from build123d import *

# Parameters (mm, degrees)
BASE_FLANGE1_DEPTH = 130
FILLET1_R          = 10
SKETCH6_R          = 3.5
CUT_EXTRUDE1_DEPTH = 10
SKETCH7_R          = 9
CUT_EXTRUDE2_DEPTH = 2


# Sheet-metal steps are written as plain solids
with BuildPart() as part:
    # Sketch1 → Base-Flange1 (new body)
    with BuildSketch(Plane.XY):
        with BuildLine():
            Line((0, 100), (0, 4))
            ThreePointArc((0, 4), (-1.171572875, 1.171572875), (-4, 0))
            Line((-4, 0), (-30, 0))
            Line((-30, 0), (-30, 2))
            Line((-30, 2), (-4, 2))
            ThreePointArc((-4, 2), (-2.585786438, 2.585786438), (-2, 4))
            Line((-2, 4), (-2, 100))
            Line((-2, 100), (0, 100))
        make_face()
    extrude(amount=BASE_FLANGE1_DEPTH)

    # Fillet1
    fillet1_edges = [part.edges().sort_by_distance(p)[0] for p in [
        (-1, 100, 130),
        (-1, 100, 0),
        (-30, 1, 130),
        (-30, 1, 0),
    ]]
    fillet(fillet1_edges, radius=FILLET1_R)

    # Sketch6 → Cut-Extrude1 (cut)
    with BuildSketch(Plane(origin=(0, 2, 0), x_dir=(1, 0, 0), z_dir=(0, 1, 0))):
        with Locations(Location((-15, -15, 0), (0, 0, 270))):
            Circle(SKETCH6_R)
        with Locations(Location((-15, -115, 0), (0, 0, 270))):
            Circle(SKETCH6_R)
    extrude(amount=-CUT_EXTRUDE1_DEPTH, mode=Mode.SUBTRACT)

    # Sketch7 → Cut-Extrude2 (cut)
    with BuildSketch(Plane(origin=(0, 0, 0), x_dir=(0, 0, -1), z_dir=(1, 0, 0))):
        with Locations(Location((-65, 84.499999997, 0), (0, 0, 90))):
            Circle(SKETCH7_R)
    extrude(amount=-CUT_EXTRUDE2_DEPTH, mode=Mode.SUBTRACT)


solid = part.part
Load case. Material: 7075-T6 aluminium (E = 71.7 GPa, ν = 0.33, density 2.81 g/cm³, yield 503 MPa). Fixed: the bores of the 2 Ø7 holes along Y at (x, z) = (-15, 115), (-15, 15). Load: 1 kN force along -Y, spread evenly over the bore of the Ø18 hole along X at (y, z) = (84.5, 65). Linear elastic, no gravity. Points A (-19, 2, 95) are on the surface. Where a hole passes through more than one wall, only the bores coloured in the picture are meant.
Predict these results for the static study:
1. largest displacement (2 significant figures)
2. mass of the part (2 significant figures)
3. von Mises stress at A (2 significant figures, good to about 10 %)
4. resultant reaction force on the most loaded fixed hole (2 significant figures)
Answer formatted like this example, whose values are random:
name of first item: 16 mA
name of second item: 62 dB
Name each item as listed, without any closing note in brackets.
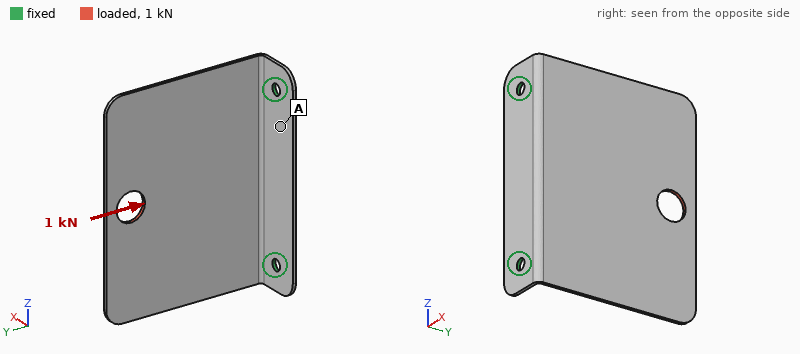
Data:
largest displacement: 1.9 mm
mass of the part: 90 g
von Mises stress at A: 38 MPa
resultant reaction force on the most loaded fixed hole: 510 N
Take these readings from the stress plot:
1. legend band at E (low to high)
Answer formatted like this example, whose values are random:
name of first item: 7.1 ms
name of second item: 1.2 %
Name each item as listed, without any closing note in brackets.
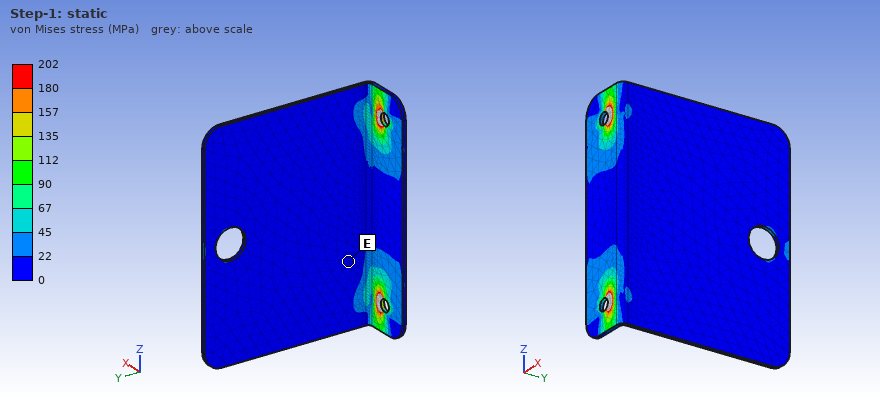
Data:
legend band at E: 0 to 22 MPa
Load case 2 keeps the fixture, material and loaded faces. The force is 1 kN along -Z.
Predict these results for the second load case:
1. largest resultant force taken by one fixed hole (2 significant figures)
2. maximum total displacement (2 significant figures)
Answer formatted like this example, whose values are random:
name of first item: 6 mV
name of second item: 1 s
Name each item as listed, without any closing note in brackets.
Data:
largest resultant force taken by one fixed hole: 970 N
maximum total displacement: 1.3 mm
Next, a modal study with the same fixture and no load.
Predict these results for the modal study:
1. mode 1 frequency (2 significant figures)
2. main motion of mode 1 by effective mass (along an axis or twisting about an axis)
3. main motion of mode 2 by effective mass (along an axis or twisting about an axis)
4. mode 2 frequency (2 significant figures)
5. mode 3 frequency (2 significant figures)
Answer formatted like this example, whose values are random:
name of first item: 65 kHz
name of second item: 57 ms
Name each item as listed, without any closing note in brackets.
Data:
mode 1 frequency: 130 Hz
main motion of mode 1 by effective mass: along X
main motion of mode 2 by effective mass: twisting about Y
mode 2 frequency: 310 Hz
mode 3 frequency: 800 Hz
